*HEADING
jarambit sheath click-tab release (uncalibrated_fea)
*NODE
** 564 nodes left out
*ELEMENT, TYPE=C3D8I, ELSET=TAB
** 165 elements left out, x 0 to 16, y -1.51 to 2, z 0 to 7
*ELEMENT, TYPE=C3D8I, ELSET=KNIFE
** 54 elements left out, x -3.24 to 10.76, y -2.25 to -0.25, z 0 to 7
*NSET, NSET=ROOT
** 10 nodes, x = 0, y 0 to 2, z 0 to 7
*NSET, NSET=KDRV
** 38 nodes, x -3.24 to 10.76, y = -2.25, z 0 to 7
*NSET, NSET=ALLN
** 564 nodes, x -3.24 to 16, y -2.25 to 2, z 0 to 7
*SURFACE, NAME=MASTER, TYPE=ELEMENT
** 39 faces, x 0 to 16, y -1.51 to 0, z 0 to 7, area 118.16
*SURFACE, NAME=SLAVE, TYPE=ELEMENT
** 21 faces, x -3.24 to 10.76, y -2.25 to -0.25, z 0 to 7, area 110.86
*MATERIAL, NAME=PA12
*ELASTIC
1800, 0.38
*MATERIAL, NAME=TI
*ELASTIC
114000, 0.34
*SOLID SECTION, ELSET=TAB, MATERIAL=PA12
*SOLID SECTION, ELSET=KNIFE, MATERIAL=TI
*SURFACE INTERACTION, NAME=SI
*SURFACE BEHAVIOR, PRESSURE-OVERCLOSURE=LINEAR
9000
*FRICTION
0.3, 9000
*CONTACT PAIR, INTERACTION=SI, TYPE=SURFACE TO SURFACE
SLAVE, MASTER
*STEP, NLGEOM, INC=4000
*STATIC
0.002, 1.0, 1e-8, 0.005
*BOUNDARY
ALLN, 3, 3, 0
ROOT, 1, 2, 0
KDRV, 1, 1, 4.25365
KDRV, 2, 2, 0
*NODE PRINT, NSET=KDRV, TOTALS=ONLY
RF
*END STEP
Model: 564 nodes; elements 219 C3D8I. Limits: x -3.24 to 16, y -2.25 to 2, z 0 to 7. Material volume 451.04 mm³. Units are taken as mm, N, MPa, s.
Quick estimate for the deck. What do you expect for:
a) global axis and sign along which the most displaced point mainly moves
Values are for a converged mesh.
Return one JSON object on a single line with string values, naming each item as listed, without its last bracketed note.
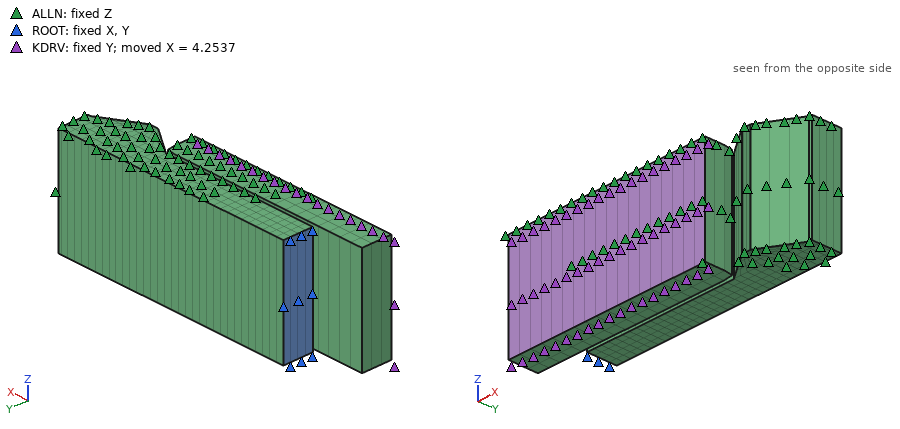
{"global axis and sign along which the most displaced point mainly moves": "+X"}
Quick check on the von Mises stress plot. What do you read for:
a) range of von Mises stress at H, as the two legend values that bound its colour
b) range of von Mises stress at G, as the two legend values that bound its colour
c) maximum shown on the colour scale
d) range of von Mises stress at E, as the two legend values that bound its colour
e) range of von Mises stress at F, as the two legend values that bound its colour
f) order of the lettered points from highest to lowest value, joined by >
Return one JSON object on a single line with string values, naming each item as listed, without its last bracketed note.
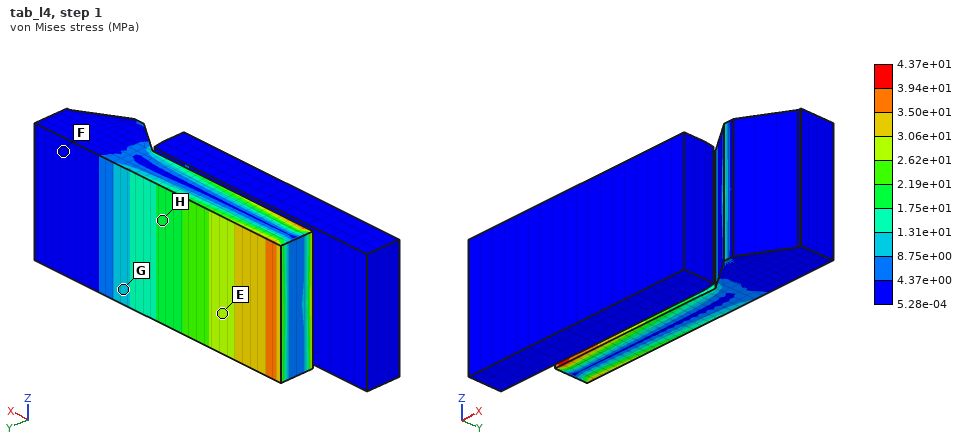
{"range of von Mises stress at H, as the two legend values that bound its colour": "1.75e+01 to 2.19e+01 MPa", "range of von Mises stress at G, as the two legend values that bound its colour": "8.75e+00 to 1.31e+01 MPa", "maximum shown on the colour scale": "4.37e+01 MPa", "range of von Mises stress at E, as the two legend values that bound its colour": "2.62e+01 to 3.06e+01 MPa", "range of von Mises stress at F, as the two legend values that bound its colour": "5.28e-04 to 4.37e+00 MPa", "order of the lettered points from highest to lowest value, joined by >": "E > H > G > F"}
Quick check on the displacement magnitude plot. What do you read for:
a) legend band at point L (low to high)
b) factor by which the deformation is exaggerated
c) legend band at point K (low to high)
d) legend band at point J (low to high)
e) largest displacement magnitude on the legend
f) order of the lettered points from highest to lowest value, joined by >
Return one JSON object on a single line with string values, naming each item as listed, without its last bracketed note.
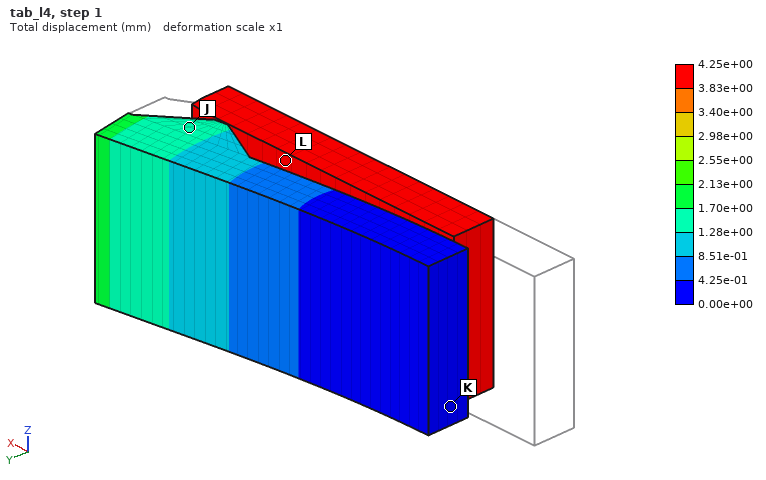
{"legend band at point L": "3.83e+00 to 4.25e+00 mm", "factor by which the deformation is exaggerated": "1", "legend band at point K": "0.00e+00 to 4.25e-01 mm", "legend band at point J": "1.28e+00 to 1.70e+00 mm", "largest displacement magnitude on the legend": "4.25e+00 mm", "order of the lettered points from highest to lowest value, joined by >": "L > J > K"}
